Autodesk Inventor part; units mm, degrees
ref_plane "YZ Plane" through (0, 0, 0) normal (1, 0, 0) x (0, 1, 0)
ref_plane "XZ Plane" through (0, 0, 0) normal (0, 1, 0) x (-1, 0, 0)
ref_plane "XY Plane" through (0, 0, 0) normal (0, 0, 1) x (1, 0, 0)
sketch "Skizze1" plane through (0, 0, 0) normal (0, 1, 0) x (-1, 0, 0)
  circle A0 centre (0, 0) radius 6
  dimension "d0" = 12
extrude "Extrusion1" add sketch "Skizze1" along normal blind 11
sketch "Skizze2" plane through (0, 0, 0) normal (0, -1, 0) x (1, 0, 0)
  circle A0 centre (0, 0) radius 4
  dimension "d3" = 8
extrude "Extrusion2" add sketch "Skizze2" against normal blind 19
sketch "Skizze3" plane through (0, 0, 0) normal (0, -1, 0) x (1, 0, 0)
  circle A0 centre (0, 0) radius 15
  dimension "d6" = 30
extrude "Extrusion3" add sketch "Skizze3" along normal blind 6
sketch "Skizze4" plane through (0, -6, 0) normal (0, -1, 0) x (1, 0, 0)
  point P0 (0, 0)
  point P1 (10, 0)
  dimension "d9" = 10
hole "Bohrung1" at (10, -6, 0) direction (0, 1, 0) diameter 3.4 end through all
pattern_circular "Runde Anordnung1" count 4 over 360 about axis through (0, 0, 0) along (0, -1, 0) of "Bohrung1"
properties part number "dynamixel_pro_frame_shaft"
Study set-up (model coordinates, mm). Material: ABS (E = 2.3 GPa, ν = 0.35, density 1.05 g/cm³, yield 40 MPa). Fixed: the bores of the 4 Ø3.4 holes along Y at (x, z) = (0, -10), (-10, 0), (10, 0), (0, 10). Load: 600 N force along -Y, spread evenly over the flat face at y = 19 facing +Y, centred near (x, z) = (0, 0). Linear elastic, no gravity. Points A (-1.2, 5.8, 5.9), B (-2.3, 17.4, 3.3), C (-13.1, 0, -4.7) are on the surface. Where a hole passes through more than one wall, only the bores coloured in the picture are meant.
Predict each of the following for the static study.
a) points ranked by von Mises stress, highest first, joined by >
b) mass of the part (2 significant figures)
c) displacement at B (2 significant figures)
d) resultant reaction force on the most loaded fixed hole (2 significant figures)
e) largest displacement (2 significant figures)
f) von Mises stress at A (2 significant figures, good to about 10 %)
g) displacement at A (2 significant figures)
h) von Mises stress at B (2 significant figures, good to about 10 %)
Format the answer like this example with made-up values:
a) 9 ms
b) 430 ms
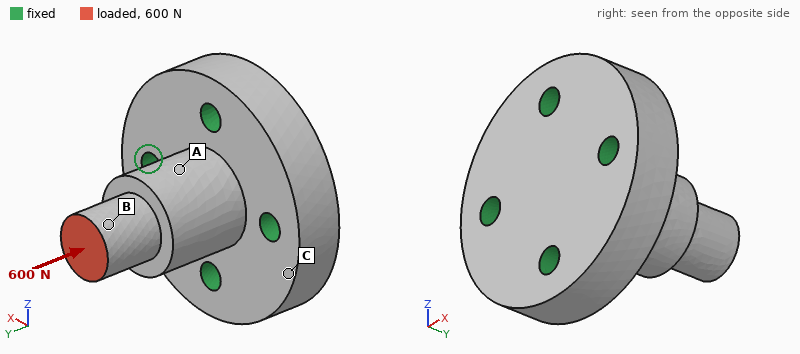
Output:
a) B > A > C
b) 6.0 g
c) 85 µm
d) 160 N
e) 93 µm
f) 4.6 MPa
g) 35 µm
h) 12 MPa
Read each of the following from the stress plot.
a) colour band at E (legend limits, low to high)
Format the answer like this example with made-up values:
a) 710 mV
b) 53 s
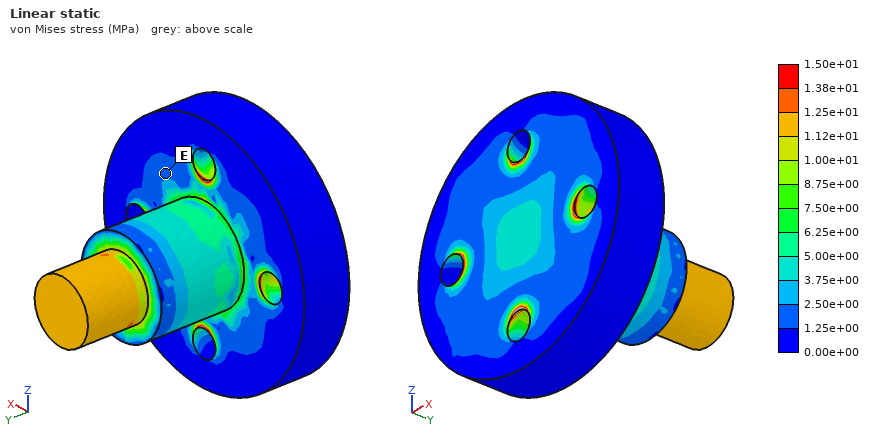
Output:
a) 1.25e+00 to 2.50e+00 MPa
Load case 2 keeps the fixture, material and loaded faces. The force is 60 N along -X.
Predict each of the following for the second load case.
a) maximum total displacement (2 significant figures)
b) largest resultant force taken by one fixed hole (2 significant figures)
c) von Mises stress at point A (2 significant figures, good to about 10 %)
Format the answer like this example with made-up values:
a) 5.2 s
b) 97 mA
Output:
a) 0.14 mm
b) 72 N
c) 1.3 MPa
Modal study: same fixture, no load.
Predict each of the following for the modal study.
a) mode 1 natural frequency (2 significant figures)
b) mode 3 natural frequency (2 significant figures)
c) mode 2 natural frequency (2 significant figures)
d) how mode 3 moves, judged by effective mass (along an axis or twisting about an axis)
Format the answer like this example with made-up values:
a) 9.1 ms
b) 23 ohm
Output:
a) 5900 Hz
b) 14 kHz
c) 5900 Hz
d) along Y
